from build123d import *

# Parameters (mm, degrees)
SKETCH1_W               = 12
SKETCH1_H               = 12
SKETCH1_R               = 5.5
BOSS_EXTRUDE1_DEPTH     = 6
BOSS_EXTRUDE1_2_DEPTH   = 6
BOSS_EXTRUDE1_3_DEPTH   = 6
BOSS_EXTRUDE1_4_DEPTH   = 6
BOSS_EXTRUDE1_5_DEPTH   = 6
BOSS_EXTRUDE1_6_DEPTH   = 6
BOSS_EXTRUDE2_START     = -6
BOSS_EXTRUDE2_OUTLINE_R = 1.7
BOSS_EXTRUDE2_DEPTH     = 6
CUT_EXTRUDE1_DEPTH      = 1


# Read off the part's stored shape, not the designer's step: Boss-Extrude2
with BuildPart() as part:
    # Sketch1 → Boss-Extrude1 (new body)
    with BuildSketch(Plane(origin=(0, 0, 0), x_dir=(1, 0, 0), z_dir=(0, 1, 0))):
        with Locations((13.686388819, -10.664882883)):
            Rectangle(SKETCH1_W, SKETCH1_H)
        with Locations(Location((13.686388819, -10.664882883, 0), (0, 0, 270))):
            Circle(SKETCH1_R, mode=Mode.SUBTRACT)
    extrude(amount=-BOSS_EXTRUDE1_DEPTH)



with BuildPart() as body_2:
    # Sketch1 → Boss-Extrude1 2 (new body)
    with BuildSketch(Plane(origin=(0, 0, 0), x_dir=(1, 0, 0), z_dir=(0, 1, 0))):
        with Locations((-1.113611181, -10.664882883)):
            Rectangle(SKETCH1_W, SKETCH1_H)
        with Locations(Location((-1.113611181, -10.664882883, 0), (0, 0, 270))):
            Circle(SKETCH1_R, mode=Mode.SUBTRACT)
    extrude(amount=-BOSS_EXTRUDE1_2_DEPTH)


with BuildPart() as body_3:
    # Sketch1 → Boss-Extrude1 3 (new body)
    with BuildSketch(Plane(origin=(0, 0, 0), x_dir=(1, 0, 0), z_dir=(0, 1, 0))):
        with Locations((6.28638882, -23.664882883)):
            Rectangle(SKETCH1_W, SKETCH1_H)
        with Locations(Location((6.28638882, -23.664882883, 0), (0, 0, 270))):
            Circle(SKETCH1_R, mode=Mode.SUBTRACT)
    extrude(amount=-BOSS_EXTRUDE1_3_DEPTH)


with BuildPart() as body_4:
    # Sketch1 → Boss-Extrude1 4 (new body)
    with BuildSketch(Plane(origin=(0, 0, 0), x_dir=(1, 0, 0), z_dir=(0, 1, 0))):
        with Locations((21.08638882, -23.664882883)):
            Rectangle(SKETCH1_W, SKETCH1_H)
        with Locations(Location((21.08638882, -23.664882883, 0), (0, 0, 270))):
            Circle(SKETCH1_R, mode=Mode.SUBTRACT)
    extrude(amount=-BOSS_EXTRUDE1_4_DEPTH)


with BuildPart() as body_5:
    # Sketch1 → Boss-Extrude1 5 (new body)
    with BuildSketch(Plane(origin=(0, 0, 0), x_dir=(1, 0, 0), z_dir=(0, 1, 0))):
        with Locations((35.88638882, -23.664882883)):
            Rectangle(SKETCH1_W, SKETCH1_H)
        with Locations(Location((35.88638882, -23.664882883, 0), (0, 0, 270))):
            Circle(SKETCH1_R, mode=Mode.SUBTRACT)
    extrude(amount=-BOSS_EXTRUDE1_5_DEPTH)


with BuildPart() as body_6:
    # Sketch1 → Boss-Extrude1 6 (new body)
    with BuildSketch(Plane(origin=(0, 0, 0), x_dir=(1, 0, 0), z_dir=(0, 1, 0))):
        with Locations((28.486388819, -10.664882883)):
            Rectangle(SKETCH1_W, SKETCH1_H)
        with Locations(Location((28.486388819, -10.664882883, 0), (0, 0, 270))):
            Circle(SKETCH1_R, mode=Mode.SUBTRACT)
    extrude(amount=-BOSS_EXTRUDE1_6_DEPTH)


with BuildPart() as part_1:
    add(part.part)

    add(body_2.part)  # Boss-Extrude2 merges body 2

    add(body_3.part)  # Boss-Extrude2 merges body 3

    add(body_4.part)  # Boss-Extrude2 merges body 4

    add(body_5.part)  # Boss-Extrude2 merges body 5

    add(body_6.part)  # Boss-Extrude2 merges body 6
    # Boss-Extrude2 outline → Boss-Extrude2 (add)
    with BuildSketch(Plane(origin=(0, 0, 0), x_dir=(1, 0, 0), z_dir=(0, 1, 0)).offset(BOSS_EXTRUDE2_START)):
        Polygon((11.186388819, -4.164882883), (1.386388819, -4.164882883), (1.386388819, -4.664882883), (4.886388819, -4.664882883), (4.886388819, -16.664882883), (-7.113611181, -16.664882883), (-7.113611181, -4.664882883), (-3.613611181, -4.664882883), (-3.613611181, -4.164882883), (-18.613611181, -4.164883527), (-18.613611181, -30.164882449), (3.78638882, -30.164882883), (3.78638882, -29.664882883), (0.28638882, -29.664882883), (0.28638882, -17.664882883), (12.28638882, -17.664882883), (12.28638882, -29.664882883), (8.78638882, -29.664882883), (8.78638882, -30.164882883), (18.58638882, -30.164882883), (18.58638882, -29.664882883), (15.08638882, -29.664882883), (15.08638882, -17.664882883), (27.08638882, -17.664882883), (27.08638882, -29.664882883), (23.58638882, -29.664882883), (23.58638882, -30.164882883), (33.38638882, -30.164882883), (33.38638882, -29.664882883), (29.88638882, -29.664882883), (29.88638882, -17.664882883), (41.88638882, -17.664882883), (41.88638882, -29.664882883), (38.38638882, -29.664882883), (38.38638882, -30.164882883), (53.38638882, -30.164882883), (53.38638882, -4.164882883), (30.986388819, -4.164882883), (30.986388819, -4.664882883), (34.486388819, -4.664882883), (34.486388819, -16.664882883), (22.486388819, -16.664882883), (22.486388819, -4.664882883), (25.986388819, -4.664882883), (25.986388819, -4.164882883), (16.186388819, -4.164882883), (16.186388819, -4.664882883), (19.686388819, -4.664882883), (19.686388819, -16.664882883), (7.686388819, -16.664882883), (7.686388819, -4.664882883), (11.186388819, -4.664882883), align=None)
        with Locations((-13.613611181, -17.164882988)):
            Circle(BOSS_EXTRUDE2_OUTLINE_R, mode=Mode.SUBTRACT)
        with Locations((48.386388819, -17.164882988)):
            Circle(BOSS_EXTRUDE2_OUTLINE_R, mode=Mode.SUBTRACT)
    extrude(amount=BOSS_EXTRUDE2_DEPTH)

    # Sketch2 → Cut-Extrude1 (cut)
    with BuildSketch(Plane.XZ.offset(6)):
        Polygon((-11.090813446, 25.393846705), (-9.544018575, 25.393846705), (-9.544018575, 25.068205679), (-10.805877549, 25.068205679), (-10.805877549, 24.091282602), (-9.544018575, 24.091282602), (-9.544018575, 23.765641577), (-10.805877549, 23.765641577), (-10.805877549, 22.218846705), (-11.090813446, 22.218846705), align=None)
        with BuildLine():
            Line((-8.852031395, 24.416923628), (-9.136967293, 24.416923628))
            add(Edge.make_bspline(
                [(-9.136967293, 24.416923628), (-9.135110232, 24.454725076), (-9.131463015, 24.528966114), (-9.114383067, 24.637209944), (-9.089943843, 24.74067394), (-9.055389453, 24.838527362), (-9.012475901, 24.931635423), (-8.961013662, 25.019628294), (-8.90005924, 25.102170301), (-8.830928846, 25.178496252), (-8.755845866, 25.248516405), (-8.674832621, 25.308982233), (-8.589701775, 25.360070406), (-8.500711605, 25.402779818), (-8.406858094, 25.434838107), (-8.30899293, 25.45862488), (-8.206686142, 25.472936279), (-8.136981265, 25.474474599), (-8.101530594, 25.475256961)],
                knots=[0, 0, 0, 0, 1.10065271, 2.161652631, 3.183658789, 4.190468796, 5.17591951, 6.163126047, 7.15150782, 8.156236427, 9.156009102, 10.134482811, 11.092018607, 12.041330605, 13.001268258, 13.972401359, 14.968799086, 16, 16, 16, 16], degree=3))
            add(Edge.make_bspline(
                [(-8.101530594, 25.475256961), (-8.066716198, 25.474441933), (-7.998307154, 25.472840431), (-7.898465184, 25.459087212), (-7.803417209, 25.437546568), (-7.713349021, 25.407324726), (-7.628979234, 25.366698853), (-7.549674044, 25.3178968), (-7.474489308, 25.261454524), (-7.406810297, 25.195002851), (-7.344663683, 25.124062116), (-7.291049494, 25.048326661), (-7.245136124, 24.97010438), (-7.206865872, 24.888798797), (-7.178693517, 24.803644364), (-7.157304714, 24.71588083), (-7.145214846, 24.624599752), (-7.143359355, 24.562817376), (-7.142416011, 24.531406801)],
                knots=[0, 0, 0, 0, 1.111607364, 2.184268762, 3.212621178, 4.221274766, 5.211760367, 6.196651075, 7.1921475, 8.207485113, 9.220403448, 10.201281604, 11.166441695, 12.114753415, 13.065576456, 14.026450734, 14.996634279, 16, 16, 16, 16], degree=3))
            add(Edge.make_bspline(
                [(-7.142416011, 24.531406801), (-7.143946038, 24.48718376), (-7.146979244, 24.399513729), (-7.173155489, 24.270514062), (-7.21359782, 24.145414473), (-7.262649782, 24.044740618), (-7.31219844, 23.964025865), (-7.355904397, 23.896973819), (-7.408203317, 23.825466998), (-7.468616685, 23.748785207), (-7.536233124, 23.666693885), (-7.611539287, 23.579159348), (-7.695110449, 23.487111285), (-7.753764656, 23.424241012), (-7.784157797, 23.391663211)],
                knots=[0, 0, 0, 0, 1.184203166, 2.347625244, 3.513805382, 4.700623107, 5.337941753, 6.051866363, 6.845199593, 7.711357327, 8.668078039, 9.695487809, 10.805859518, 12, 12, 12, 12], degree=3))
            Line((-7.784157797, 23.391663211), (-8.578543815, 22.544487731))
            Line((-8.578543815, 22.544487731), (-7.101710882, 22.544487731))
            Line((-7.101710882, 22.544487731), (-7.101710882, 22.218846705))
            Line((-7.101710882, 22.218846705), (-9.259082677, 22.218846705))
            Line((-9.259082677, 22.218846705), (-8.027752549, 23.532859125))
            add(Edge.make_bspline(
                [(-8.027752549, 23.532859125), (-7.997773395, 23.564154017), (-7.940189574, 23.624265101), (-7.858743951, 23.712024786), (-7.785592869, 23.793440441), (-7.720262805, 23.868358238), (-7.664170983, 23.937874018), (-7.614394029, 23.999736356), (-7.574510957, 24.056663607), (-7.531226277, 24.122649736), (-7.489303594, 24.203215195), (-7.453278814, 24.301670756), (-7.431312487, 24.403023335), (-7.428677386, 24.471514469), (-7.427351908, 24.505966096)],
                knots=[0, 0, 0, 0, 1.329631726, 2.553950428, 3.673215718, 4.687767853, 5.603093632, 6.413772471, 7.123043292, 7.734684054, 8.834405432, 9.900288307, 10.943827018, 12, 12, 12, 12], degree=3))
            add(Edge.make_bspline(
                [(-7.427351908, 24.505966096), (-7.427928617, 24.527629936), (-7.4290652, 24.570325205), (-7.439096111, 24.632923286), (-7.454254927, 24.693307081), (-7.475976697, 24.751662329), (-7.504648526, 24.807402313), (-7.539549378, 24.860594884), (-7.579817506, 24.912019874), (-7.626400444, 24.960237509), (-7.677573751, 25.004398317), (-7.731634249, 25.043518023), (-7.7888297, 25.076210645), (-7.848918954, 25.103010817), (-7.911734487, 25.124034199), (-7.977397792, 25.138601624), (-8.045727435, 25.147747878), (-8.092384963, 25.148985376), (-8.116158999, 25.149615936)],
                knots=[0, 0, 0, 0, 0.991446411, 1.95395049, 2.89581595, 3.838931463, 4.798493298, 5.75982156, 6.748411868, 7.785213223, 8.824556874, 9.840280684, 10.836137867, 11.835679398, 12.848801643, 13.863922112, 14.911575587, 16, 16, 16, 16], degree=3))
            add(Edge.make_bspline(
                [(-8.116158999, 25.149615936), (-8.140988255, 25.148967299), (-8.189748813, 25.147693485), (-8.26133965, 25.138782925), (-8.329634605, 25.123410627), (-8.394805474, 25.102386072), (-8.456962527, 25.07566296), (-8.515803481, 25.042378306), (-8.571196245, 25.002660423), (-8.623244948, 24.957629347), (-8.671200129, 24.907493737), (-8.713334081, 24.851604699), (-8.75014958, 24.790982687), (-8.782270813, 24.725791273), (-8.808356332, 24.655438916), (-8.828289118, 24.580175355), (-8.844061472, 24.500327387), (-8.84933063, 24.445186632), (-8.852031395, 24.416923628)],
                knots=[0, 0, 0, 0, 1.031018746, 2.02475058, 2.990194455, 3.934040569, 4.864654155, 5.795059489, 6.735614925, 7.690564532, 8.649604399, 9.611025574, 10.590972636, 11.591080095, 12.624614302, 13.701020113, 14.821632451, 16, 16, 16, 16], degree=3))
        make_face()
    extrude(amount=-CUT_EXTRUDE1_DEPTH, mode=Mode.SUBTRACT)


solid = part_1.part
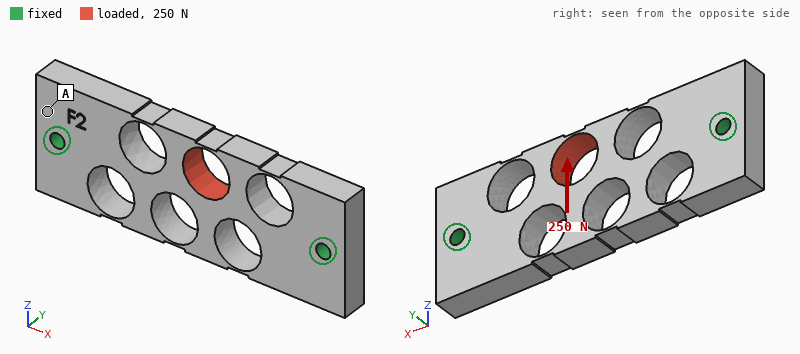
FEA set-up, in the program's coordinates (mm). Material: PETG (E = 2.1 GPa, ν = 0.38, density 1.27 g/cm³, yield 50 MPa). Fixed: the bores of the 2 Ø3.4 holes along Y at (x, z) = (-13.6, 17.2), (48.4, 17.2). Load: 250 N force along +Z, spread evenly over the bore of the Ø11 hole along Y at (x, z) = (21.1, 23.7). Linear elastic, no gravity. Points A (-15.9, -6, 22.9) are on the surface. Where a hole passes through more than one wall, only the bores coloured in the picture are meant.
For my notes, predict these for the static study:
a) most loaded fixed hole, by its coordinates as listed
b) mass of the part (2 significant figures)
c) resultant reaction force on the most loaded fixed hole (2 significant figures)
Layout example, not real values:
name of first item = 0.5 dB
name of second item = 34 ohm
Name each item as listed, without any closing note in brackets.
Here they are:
most loaded fixed hole, by its coordinates as listed = (48.4, 17.2)
mass of the part = 9.7 g
resultant reaction force on the most loaded fixed hole = 150 N
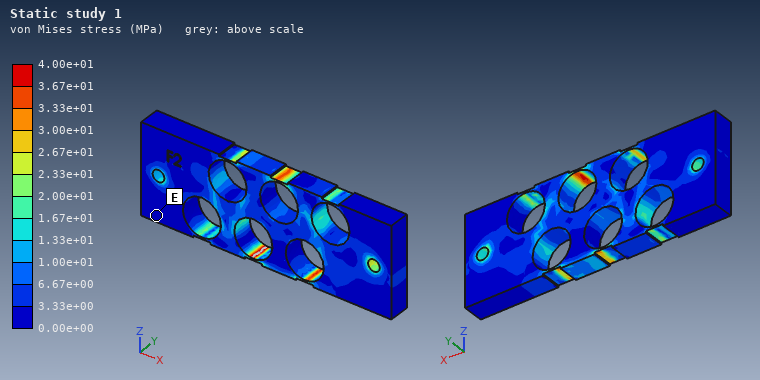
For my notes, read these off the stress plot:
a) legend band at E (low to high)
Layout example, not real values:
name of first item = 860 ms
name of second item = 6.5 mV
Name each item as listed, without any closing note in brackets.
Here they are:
legend band at E = 0.00e+00 to 3.33e+00 MPa
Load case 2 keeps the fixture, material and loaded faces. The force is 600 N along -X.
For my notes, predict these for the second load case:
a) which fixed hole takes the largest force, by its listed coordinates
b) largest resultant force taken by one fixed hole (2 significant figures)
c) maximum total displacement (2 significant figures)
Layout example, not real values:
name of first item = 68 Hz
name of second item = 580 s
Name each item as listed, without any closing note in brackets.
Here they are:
which fixed hole takes the largest force, by its listed coordinates = (48.4, 17.2)
largest resultant force taken by one fixed hole = 340 N
maximum total displacement = 0.19 mm
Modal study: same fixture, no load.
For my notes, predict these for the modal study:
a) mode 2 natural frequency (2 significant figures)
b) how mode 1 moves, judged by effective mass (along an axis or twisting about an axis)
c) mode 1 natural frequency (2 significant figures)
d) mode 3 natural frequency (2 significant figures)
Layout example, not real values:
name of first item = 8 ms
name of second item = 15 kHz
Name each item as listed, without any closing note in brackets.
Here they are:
mode 2 natural frequency = 2400 Hz
how mode 1 moves, judged by effective mass = along Y
mode 1 natural frequency = 1800 Hz
mode 3 natural frequency = 2500 Hz
